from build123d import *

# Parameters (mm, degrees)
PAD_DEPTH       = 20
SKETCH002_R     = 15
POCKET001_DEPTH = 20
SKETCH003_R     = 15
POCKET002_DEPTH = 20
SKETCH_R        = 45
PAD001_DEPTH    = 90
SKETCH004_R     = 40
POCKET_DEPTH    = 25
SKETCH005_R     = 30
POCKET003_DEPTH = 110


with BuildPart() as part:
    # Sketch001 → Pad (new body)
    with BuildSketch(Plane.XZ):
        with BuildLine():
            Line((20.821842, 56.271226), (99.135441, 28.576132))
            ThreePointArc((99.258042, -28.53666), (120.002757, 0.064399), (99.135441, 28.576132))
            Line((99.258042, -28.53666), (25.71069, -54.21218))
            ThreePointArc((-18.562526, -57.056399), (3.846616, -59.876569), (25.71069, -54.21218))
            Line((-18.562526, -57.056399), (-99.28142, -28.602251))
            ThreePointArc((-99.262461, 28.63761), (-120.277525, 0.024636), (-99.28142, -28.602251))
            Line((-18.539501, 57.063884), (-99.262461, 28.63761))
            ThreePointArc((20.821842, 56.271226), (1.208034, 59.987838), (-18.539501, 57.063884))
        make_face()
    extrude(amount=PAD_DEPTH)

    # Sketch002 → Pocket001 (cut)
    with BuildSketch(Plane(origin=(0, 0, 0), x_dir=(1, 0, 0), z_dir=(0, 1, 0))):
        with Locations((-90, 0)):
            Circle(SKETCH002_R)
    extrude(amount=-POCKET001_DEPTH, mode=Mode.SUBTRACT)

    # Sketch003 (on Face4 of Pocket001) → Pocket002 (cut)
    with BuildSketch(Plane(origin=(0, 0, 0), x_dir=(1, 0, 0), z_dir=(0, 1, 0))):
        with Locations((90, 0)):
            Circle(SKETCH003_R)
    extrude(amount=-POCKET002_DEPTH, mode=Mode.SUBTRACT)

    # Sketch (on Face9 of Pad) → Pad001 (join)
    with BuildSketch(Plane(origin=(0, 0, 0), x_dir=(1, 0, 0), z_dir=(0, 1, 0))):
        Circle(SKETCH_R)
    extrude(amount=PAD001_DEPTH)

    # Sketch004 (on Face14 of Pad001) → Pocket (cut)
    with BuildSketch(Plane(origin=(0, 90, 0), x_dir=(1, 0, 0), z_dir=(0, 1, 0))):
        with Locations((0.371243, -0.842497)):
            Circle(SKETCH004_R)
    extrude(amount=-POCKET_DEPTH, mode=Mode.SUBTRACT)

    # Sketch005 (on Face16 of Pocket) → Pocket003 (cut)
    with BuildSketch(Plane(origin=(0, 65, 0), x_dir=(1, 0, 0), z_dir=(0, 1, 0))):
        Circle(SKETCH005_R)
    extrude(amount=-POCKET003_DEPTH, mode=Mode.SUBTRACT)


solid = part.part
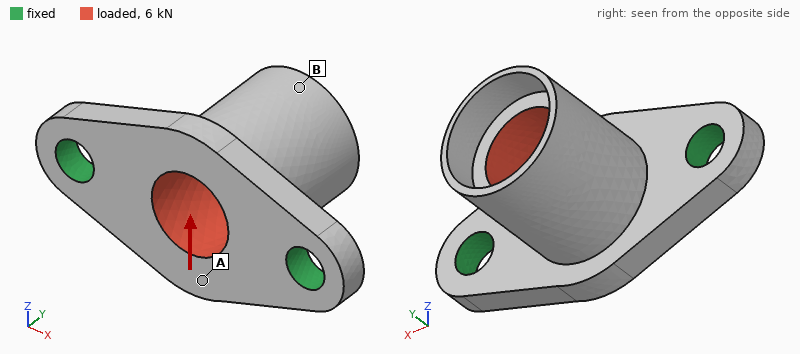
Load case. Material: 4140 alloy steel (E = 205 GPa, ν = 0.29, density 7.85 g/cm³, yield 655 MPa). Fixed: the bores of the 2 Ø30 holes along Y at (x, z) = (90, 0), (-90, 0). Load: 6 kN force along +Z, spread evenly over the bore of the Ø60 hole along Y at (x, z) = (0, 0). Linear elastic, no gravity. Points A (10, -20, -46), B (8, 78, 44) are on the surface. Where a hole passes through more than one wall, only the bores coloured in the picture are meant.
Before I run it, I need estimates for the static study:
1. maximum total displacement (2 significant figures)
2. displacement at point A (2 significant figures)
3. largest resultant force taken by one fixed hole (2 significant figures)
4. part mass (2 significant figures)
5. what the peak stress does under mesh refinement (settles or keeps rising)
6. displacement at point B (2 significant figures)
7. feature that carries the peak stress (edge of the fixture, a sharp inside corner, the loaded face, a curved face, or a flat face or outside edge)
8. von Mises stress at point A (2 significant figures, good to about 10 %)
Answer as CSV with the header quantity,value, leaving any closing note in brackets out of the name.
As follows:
quantity,value
maximum total displacement,29 µm
displacement at point A,11 µm
largest resultant force taken by one fixed hole,3.0 kN
part mass,4.5 kg
what the peak stress does under mesh refinement,keeps rising
displacement at point B,27 µm
feature that carries the peak stress,edge of the fixture
von Mises stress at point A,7.1 MPa
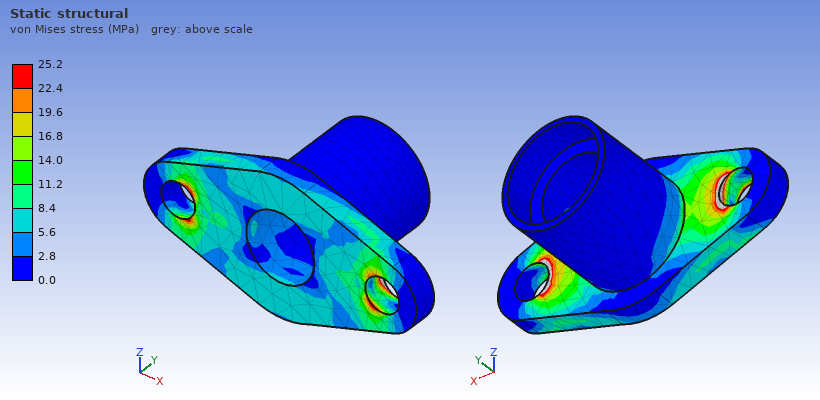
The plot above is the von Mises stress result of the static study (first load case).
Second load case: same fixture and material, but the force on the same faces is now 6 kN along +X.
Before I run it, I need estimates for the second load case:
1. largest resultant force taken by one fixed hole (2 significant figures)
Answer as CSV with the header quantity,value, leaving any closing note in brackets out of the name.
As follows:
quantity,value
largest resultant force taken by one fixed hole,3.4 kN
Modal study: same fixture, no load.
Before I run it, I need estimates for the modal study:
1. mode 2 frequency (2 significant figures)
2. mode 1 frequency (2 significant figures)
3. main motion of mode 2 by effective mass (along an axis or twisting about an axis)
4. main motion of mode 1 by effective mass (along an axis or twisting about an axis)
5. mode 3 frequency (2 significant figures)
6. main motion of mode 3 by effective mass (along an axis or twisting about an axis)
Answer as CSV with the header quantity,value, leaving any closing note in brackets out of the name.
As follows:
quantity,value
mode 2 frequency,2800 Hz
mode 1 frequency,1400 Hz
main motion of mode 2 by effective mass,along Y
main motion of mode 1 by effective mass,along Z
mode 3 frequency,3300 Hz
main motion of mode 3 by effective mass,along X
